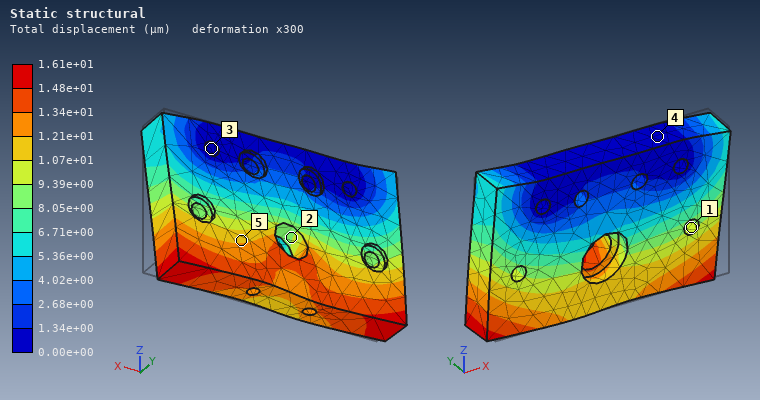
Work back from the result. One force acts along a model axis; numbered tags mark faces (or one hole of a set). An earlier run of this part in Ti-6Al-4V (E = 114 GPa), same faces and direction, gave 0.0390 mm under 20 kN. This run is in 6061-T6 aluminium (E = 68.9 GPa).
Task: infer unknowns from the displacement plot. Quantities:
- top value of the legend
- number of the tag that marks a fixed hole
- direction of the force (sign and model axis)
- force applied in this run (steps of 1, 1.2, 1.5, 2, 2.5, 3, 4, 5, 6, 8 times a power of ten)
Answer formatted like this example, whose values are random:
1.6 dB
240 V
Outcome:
1.61e+01 µm
3
-X
5 kN
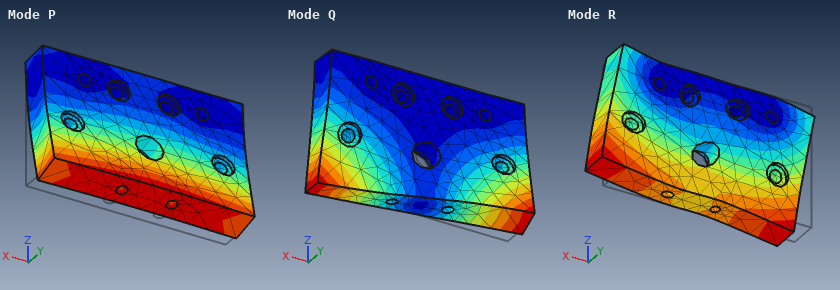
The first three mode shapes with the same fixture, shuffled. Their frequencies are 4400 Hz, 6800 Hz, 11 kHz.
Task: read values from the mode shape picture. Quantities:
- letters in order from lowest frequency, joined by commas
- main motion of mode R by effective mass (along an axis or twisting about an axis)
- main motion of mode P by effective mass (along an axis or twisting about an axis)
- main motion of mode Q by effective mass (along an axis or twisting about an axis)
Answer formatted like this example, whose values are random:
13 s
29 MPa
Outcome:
P, Q, R
along X
along Y
twisting about Z
